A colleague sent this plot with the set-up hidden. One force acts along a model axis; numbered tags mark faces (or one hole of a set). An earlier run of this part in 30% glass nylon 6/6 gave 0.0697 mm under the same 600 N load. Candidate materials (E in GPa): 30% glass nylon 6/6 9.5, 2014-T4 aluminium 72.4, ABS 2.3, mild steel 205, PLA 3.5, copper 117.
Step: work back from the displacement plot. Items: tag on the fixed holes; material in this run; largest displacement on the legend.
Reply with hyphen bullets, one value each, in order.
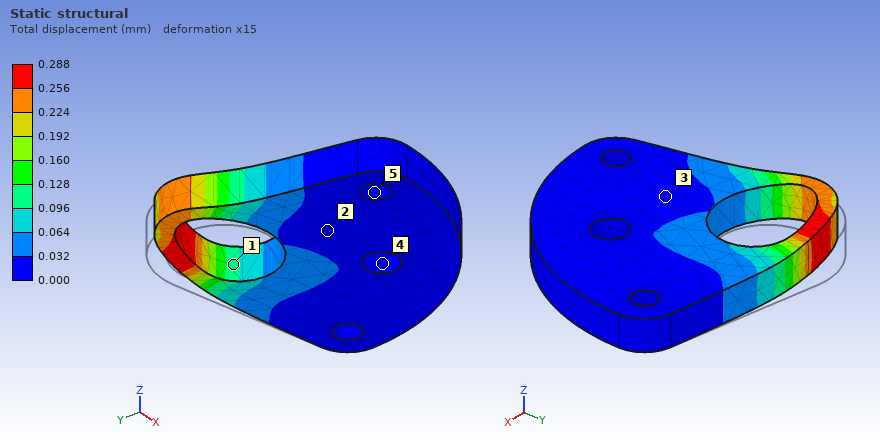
- 5
- ABS
- 0.288 mm
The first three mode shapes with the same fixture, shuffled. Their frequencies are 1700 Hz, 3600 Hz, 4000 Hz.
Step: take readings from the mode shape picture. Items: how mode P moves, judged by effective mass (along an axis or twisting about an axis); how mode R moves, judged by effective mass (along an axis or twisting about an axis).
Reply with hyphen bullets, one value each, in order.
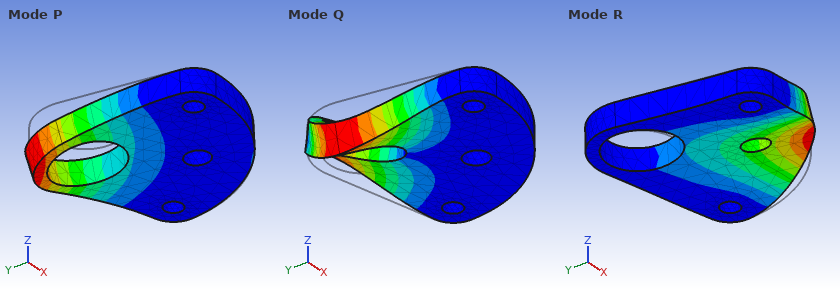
- along Z
- along Z
